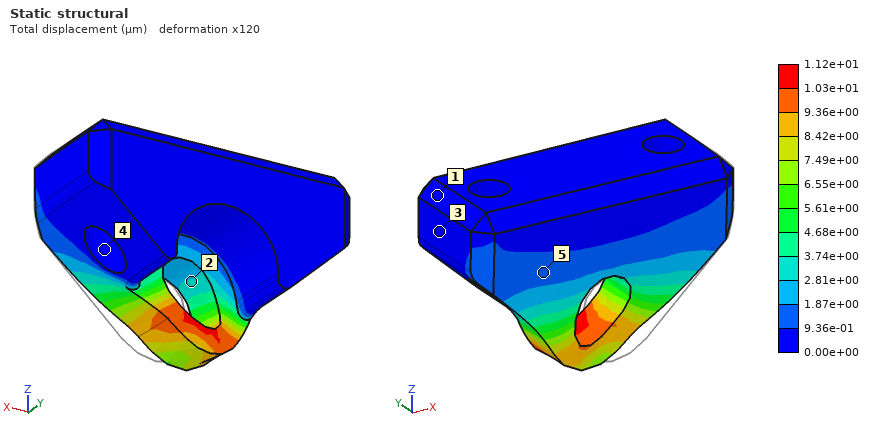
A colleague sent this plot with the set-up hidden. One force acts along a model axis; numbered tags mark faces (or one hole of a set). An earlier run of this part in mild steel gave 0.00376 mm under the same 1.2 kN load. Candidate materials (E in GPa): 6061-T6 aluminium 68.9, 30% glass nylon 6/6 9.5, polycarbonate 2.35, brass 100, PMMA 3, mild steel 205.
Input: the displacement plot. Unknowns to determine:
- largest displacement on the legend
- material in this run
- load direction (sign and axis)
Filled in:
1.12e+01 µm
6061-T6 aluminium
-X
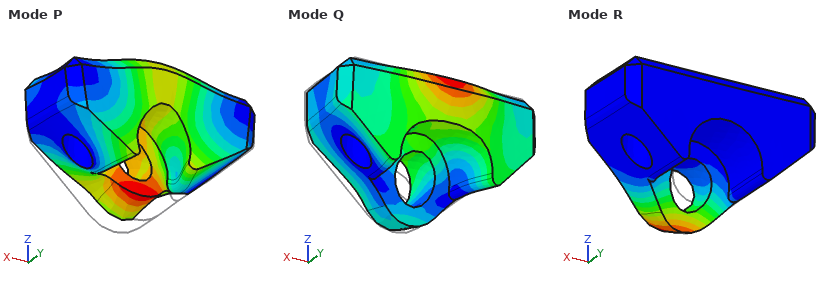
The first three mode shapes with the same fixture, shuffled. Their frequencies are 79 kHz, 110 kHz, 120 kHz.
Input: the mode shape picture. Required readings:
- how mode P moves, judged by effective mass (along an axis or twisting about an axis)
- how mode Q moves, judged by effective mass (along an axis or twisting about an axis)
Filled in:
along Z
along Y
